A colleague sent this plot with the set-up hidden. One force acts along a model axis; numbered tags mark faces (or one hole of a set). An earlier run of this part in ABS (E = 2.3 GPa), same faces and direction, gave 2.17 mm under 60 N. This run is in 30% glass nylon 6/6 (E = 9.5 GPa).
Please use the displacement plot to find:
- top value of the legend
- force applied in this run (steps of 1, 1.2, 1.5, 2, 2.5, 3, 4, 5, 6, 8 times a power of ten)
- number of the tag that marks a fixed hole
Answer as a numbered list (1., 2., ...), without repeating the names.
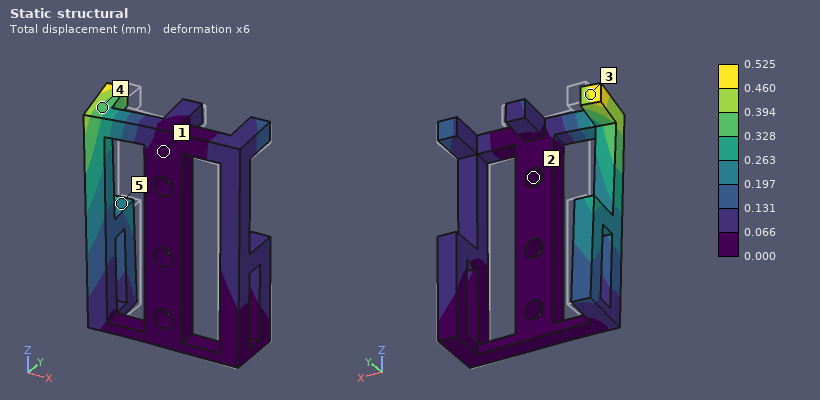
1. 0.525 mm
2. 60 N
3. 2
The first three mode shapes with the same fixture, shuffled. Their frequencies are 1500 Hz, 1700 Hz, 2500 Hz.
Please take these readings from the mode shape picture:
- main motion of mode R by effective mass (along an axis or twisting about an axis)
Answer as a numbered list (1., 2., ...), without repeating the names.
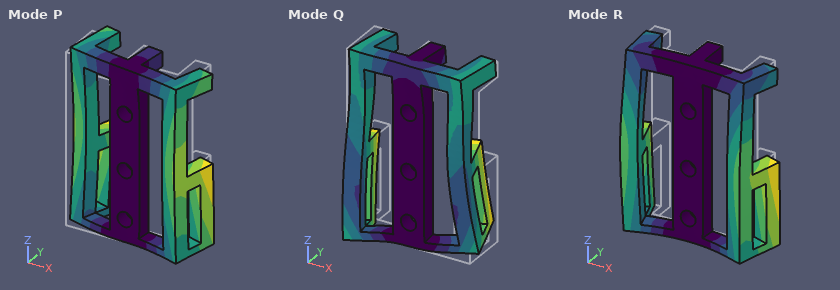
1. along Y
